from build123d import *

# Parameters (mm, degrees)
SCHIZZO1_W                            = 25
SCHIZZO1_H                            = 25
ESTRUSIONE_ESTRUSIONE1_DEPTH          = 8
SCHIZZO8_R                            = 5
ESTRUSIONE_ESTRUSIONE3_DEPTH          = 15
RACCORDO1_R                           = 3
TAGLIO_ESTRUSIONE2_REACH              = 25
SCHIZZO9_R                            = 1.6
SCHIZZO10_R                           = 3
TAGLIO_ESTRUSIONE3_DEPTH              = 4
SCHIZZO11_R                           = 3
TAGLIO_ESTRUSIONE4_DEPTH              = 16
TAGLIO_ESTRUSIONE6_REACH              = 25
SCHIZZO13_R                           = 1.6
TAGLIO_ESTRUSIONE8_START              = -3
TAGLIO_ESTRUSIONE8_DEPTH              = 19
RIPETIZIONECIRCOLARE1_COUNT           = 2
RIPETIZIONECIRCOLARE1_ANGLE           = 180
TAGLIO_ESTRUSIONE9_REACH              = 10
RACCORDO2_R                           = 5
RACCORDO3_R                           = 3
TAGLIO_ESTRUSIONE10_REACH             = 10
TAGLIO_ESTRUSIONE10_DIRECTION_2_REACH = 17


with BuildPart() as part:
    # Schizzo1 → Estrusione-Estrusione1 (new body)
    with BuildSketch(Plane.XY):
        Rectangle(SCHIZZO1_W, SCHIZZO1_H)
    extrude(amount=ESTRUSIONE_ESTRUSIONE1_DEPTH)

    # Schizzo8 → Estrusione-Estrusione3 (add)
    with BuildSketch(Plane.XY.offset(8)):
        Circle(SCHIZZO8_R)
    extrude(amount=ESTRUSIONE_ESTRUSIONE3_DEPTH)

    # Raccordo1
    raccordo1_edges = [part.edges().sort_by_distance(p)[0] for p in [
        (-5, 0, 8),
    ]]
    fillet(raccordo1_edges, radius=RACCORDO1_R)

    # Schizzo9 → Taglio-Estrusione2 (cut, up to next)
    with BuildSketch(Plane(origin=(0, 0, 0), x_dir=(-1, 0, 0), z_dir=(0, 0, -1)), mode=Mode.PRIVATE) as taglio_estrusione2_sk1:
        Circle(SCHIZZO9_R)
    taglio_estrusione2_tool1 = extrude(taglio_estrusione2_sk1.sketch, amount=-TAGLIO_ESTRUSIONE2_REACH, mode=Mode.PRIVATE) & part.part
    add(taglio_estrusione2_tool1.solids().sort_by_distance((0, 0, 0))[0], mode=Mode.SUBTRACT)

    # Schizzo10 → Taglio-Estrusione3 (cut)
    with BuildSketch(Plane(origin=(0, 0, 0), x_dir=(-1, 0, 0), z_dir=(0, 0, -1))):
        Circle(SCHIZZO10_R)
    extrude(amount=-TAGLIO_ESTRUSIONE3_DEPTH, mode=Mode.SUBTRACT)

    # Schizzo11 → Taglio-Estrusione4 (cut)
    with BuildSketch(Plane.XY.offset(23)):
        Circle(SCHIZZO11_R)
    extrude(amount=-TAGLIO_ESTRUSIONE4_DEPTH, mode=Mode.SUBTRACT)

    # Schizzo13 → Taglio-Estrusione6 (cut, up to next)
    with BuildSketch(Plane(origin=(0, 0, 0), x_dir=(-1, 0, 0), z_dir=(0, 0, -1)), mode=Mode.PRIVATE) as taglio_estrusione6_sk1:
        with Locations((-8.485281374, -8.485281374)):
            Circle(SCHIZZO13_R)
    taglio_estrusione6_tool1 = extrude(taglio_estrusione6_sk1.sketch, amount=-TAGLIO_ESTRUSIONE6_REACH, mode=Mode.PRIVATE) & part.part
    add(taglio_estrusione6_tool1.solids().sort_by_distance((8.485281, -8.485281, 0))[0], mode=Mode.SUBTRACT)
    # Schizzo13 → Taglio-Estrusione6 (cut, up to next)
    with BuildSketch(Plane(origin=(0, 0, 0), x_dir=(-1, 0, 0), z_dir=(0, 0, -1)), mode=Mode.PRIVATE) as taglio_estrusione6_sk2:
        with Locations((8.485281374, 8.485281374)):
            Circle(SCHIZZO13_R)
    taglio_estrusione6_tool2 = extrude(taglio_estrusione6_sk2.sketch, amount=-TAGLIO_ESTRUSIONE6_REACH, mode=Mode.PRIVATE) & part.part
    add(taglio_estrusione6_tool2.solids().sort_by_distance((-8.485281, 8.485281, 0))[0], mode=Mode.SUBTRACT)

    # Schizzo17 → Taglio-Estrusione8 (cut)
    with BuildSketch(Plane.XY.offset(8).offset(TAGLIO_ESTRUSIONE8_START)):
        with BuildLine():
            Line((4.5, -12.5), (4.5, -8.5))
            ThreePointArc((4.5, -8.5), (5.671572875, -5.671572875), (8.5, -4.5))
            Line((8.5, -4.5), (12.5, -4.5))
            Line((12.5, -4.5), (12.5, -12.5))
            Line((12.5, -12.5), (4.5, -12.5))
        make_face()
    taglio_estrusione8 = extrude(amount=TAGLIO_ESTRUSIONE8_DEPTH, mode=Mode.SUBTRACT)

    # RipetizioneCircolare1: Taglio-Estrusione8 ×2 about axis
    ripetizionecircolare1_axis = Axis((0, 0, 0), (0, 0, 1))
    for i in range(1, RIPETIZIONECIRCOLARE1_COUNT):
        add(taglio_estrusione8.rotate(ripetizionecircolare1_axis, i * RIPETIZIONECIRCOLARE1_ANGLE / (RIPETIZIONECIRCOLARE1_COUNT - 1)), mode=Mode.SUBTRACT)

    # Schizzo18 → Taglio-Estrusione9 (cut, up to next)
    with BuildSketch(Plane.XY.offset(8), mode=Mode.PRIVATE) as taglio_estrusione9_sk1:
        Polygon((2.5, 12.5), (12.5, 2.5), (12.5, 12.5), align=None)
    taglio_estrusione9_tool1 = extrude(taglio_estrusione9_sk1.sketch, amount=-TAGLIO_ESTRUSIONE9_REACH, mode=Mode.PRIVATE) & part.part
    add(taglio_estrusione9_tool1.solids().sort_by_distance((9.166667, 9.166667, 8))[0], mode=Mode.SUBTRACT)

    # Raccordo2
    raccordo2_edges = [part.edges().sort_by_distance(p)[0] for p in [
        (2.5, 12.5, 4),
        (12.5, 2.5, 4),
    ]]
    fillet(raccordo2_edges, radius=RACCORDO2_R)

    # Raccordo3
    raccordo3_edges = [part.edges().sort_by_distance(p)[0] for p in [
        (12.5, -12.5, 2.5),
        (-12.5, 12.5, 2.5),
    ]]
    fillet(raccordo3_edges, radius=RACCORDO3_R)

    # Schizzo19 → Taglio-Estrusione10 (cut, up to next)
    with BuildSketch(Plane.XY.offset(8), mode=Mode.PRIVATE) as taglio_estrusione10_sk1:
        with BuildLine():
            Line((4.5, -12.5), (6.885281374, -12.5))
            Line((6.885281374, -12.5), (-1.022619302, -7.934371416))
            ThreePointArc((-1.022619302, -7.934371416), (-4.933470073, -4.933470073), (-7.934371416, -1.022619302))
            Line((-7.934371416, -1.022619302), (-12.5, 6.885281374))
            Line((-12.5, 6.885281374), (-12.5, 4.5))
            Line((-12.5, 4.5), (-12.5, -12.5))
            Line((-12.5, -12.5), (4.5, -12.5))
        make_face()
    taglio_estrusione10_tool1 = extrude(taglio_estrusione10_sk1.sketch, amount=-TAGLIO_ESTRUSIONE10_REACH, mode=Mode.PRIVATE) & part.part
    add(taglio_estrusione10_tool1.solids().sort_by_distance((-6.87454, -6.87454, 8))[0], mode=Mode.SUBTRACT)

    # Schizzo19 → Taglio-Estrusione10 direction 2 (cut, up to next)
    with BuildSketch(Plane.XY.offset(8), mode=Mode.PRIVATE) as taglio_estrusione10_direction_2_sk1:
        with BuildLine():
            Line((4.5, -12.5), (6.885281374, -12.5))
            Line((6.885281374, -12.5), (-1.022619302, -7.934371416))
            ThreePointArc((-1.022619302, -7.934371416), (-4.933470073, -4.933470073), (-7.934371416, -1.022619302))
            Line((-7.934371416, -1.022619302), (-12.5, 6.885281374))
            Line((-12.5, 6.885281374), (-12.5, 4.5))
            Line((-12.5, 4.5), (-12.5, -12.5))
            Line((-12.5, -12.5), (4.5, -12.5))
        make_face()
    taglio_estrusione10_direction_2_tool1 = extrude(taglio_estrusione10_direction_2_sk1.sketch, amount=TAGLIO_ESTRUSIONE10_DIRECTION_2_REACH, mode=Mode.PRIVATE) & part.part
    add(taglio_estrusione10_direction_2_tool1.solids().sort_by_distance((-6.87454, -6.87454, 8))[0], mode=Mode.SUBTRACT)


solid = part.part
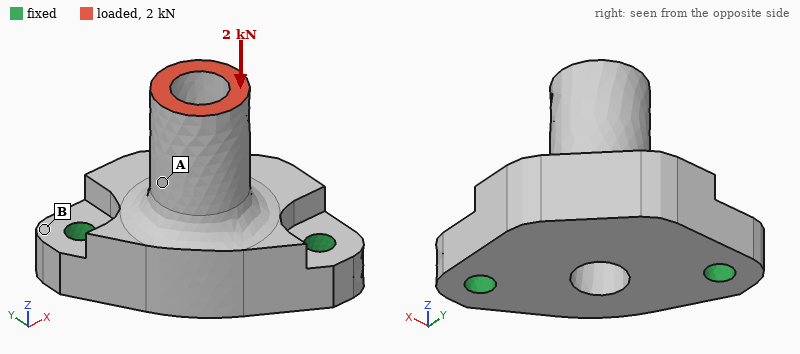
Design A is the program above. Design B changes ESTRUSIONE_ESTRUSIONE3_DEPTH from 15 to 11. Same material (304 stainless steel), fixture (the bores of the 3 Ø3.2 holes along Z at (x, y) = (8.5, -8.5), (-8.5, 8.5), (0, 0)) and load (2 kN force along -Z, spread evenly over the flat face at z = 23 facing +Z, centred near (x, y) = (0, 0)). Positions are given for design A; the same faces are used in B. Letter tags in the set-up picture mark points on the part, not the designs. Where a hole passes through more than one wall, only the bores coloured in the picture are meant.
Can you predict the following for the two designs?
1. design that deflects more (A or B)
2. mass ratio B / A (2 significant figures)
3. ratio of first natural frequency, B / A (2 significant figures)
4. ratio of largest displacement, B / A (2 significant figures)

A
0.95
1.3
0.80
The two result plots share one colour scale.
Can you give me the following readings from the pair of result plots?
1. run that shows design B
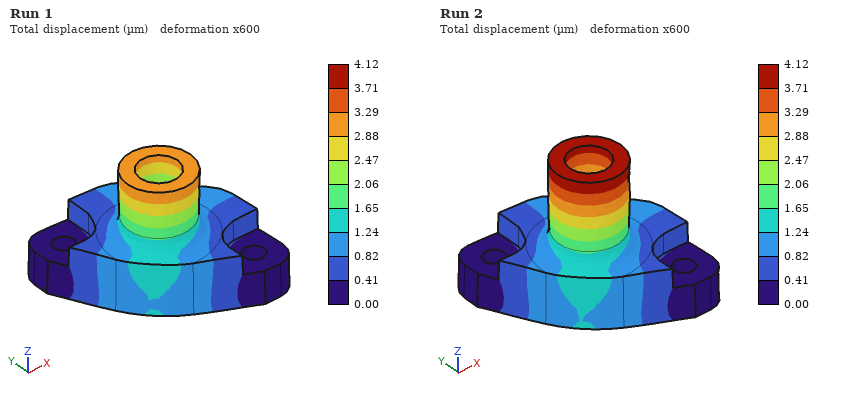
Run 1
